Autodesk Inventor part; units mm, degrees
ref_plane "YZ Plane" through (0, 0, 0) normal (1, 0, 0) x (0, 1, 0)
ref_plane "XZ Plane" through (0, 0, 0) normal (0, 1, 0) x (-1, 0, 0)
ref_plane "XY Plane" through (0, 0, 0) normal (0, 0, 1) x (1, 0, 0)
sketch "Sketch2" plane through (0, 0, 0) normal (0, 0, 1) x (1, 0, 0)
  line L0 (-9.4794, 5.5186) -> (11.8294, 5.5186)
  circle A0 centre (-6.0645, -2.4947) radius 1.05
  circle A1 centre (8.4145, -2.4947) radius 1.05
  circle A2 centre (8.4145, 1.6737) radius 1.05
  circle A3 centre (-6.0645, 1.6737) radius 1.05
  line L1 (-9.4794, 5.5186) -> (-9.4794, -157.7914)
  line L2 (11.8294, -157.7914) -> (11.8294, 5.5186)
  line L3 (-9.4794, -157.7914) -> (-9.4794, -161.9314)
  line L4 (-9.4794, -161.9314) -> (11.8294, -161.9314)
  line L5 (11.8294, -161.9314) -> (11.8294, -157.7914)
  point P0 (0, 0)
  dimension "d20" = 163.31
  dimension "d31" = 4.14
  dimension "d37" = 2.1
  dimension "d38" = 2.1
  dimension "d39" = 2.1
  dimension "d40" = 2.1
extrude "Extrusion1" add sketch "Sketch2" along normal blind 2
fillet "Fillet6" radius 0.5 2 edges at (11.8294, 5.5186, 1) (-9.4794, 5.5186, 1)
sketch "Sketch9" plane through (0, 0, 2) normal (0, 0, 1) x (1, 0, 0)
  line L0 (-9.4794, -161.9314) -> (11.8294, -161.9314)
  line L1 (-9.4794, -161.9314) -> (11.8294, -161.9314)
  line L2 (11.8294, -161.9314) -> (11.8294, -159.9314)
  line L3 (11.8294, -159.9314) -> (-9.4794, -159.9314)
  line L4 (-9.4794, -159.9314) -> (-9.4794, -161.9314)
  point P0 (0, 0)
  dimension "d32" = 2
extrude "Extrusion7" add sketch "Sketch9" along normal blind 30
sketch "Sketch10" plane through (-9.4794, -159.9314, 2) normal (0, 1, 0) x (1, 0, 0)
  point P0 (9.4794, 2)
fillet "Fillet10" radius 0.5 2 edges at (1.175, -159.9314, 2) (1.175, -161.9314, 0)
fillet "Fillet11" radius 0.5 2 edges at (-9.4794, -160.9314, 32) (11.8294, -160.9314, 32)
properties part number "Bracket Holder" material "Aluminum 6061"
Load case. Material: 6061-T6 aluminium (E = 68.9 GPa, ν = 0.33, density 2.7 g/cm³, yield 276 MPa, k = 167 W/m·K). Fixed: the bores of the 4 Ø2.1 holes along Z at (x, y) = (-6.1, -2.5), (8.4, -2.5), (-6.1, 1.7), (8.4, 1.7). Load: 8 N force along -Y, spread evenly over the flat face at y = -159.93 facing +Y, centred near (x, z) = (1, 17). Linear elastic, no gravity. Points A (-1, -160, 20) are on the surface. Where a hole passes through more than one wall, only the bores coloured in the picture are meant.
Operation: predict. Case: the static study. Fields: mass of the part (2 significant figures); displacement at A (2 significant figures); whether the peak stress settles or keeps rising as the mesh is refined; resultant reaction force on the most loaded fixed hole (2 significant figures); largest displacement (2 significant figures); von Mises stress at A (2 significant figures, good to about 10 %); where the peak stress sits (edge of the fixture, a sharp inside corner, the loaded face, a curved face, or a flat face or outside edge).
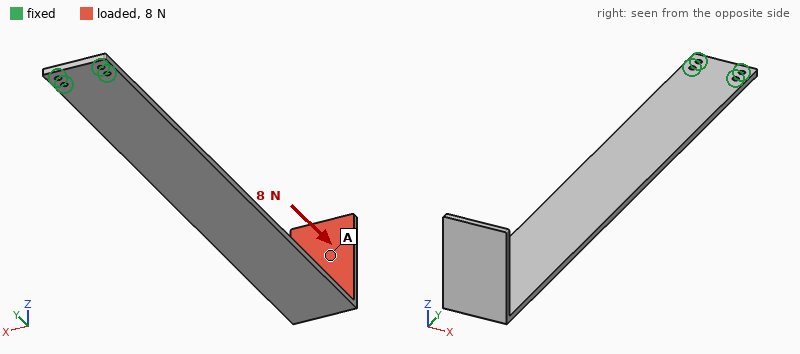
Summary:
23 g
1.7 mm
keeps rising
5.8 N
1.8 mm
1.5 MPa
edge of the fixture
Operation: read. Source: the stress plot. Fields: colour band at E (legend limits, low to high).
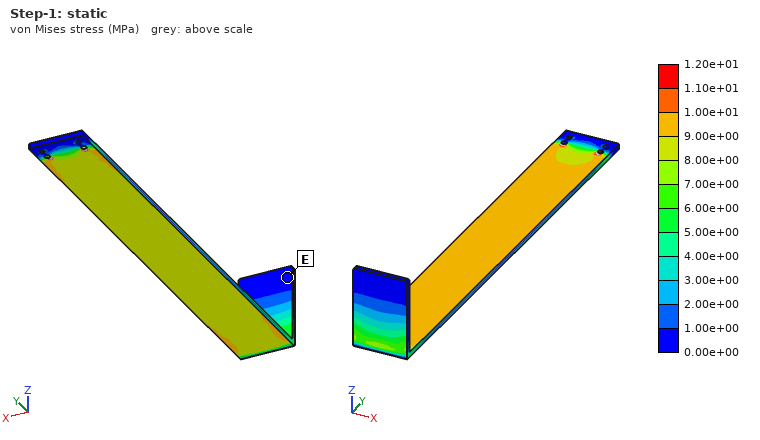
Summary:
0.00e+00 to 1.00e+00 MPa
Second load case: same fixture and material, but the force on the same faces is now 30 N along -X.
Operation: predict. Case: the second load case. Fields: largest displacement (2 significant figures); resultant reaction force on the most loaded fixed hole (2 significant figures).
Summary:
2.0 mm
260 N
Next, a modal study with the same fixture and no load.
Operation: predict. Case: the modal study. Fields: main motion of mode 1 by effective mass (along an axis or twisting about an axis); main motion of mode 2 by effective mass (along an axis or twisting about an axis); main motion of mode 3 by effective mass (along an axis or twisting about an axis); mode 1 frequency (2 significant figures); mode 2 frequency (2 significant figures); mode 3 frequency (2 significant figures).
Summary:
along Z
along Z
along X
48 Hz
310 Hz
360 Hz
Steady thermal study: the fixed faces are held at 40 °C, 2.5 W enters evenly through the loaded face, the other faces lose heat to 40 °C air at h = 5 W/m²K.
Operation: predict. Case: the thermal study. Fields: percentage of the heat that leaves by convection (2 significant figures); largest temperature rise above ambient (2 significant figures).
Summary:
36 %
46 K
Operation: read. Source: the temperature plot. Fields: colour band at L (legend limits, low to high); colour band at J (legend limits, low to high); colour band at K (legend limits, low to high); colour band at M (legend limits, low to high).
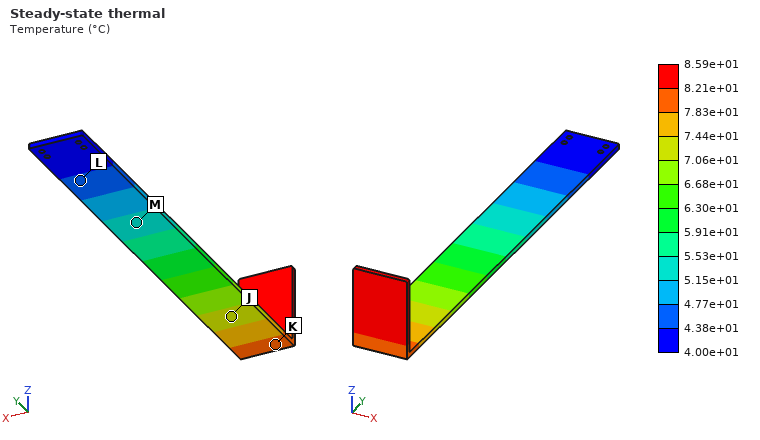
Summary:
4.38e+01 to 4.77e+01 °C
7.06e+01 to 7.44e+01 °C
7.83e+01 to 8.21e+01 °C
5.15e+01 to 5.53e+01 °C
